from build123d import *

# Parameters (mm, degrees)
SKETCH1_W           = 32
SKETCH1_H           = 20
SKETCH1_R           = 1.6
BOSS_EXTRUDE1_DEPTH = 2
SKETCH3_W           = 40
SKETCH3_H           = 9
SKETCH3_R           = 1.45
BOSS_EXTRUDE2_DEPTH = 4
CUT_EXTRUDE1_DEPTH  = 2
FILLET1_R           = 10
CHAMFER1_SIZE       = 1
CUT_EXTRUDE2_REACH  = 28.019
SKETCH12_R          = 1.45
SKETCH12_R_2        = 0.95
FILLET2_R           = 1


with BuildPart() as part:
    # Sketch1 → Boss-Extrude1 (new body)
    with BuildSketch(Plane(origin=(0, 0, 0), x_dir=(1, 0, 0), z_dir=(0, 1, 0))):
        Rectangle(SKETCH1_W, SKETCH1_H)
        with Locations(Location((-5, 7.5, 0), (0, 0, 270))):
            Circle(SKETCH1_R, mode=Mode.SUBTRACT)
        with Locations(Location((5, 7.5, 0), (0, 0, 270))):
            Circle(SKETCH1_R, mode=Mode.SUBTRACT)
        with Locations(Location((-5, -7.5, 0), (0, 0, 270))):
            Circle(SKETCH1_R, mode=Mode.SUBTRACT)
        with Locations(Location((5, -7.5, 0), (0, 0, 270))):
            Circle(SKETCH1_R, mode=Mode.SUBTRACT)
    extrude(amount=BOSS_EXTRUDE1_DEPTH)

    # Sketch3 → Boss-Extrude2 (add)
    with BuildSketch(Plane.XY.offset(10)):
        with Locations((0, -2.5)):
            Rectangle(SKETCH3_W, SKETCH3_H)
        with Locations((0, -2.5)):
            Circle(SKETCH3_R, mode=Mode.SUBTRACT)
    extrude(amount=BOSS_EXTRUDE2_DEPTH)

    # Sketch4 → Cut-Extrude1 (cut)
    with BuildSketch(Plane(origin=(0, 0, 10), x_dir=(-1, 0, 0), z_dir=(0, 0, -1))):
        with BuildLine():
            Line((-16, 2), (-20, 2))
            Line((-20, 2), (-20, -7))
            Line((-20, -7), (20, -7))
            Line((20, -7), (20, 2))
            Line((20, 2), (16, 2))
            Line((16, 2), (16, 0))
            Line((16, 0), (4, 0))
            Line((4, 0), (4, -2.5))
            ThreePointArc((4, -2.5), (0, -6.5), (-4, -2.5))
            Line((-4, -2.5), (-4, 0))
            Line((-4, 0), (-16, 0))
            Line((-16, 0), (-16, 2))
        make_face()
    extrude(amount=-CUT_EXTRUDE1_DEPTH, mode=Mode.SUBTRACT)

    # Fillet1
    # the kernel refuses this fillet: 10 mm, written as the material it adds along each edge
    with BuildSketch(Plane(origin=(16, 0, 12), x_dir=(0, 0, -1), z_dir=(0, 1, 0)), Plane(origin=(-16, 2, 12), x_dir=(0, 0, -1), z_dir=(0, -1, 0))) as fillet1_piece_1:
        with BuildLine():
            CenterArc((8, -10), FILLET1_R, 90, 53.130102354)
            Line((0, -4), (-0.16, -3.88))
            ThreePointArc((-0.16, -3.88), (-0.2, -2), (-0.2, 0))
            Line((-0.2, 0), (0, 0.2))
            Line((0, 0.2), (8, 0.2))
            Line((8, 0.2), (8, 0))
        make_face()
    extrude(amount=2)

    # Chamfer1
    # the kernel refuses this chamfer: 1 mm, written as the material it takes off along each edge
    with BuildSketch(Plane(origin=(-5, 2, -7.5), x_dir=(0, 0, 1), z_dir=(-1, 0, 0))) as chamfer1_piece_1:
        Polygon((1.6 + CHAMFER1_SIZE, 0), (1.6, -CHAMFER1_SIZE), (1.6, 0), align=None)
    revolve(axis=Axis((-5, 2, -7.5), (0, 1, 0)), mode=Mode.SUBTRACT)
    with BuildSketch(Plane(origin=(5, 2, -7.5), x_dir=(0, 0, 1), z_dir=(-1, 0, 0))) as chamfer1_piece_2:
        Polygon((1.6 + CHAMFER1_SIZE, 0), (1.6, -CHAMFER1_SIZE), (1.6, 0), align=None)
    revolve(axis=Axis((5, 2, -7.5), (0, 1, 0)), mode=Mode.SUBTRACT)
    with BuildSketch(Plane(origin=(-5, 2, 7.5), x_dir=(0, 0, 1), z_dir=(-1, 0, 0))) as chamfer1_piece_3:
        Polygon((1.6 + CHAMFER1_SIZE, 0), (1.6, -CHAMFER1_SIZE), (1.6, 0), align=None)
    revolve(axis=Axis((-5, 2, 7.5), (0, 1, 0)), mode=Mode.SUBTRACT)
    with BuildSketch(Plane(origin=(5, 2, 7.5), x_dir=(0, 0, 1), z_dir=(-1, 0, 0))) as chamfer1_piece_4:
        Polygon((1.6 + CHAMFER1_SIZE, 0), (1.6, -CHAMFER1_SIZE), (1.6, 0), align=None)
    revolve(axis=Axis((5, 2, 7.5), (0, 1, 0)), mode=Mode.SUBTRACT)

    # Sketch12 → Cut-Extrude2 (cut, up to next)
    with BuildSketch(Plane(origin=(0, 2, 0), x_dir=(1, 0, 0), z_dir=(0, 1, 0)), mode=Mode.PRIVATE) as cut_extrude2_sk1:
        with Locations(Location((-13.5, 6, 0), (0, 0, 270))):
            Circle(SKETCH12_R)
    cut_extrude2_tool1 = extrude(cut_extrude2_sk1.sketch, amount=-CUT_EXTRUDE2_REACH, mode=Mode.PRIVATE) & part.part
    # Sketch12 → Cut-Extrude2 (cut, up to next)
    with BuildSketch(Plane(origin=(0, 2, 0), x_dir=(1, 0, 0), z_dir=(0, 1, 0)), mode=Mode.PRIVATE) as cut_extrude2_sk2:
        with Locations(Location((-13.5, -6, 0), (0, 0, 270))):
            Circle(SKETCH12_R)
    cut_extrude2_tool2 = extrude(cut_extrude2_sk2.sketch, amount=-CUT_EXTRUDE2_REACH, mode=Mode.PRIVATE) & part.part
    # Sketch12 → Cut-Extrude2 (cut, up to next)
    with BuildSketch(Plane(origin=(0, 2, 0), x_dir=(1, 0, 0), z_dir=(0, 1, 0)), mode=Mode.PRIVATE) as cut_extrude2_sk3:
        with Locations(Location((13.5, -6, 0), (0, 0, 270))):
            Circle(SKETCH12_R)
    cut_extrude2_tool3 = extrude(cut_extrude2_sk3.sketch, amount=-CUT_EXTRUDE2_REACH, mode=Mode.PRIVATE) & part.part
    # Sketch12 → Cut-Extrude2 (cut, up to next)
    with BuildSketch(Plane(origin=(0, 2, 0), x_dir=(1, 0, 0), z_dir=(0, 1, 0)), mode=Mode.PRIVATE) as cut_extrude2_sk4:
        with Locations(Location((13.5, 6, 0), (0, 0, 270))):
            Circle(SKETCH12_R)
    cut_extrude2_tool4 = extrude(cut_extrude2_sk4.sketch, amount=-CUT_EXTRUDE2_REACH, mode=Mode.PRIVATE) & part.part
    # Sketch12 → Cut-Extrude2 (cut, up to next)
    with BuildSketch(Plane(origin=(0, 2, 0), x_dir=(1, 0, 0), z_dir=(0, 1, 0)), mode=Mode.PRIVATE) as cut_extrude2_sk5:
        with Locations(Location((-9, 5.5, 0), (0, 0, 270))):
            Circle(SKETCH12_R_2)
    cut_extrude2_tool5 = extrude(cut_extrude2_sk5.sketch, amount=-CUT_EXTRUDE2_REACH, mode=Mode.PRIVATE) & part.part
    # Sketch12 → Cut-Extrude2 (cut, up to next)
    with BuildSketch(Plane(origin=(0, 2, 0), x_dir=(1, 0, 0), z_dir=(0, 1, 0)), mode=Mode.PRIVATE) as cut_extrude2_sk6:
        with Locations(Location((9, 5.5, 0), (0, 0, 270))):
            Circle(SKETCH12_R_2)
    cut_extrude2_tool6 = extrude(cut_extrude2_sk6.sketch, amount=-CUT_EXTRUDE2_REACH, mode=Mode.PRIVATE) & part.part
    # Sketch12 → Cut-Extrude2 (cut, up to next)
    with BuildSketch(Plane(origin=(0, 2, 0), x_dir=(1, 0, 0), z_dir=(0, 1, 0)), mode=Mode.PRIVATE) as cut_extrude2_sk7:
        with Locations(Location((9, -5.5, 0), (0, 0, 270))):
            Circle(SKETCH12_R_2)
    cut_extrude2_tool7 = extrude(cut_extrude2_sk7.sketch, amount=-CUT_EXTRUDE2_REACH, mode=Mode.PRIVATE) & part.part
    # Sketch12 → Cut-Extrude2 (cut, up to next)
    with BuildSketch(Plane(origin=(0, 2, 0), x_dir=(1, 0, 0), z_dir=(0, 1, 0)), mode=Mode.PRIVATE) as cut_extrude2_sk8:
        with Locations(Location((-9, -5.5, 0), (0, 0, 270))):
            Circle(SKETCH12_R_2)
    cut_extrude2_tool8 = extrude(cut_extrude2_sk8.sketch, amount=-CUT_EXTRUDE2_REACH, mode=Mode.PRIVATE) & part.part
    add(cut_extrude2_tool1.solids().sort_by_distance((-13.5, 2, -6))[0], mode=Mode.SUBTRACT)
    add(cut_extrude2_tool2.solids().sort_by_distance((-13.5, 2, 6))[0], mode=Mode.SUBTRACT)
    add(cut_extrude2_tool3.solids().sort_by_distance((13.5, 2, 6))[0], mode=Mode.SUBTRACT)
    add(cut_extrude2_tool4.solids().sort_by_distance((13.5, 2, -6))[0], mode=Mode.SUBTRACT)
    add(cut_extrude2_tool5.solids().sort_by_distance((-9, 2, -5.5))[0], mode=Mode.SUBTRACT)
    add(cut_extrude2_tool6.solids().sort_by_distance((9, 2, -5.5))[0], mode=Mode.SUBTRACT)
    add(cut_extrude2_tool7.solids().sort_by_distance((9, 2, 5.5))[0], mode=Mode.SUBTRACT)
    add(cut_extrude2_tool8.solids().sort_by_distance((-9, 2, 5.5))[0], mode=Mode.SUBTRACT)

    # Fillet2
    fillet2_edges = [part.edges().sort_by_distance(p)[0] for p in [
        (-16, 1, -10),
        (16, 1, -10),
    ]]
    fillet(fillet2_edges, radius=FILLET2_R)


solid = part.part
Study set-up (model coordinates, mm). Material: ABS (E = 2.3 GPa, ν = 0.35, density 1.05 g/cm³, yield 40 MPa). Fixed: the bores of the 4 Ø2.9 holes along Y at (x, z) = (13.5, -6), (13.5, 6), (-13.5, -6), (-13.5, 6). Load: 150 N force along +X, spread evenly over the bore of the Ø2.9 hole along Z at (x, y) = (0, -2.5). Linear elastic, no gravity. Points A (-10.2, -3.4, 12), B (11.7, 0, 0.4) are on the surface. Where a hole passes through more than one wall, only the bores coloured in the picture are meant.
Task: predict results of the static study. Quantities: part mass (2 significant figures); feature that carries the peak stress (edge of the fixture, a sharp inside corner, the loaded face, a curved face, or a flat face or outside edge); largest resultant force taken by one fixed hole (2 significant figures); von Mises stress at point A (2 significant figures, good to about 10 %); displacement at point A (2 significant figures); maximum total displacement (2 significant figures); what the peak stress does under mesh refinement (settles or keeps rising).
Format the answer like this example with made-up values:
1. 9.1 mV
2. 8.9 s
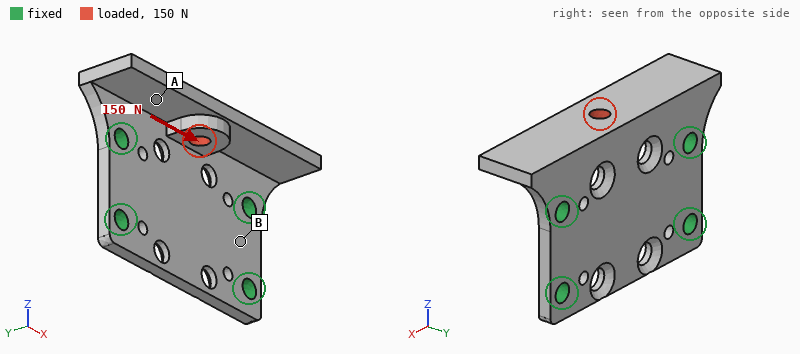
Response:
1. 2.2 g
2. edge of the fixture
3. 74 N
4. 4.4 MPa
5. 0.082 mm
6. 0.16 mm
7. keeps rising
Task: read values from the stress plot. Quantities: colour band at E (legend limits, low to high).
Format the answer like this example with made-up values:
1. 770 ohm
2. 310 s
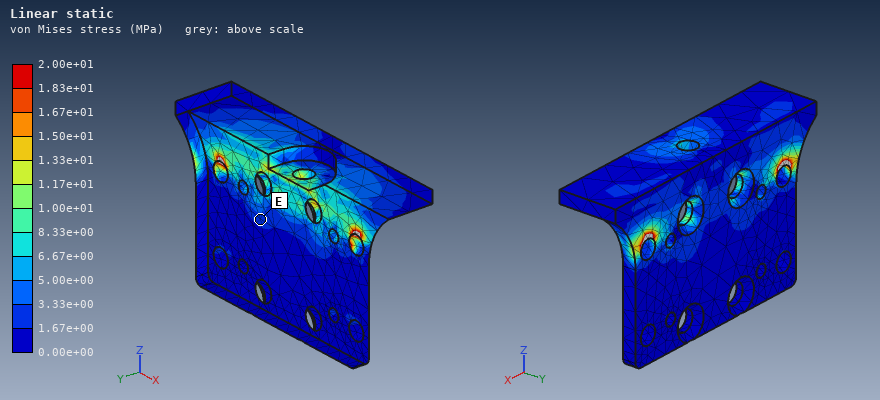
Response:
1. 1.67e+00 to 3.33e+00 MPa
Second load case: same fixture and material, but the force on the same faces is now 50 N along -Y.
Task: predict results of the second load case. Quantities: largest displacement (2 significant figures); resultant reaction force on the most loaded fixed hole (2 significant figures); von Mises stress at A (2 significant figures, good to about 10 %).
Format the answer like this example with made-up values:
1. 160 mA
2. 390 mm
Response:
1. 0.23 mm
2. 31 N
3. 3.3 MPa
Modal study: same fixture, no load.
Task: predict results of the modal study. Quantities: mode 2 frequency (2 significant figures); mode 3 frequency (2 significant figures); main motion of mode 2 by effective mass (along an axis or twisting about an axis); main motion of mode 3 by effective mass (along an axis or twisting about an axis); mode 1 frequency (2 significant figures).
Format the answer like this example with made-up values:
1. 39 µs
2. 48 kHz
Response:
1. 3600 Hz
2. 4600 Hz
3. twisting about Z
4. along Y
5. 2500 Hz
